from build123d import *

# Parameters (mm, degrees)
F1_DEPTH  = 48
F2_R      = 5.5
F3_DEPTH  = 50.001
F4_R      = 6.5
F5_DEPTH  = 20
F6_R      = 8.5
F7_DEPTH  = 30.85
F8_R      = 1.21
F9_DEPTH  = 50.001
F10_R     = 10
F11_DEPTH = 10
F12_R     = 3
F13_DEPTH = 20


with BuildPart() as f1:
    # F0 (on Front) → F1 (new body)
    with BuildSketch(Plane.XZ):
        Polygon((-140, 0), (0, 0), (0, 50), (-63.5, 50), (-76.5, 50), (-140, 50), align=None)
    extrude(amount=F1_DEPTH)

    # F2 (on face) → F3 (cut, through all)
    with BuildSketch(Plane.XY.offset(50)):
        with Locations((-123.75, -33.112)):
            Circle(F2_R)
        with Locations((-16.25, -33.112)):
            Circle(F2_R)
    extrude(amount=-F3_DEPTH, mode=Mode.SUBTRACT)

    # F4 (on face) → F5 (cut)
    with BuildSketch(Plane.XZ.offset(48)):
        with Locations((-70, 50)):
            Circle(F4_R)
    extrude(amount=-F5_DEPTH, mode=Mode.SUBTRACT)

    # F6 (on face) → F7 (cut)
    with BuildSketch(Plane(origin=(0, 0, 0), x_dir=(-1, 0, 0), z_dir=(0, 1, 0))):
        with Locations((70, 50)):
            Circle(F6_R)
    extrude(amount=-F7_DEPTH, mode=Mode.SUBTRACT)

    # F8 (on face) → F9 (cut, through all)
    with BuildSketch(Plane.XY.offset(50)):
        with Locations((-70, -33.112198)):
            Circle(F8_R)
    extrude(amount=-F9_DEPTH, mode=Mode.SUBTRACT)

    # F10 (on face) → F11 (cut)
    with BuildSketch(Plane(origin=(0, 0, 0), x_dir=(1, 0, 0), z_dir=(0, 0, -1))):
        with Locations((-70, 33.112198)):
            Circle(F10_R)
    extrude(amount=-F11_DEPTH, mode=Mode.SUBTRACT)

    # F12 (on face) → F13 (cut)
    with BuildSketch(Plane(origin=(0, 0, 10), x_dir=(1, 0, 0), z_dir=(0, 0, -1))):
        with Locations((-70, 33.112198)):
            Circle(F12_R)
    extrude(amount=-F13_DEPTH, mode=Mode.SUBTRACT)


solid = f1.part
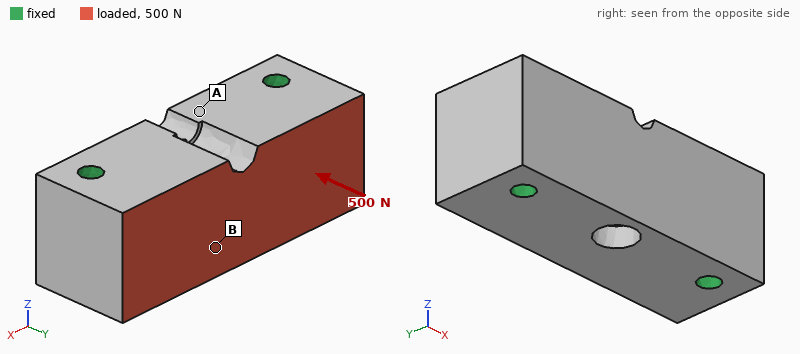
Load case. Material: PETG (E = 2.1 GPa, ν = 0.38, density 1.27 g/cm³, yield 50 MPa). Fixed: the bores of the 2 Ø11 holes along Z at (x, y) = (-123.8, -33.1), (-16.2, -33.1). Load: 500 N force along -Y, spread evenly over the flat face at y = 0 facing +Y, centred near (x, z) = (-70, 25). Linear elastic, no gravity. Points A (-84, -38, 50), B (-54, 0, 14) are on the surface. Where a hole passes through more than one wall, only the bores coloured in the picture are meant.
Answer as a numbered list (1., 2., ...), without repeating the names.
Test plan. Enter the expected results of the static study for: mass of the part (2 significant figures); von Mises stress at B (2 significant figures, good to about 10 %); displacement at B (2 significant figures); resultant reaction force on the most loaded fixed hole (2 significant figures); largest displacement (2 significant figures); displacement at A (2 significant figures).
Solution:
1. 400 g
2. 0.15 MPa
3. 5.7 µm
4. 260 N
5. 6.9 µm
6. 5.4 µm
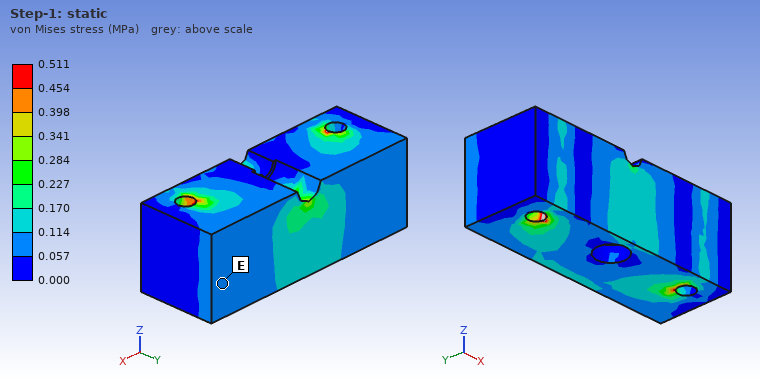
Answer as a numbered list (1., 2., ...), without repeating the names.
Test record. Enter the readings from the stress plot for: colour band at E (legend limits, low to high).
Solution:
1. 0.057 to 0.114 MPa
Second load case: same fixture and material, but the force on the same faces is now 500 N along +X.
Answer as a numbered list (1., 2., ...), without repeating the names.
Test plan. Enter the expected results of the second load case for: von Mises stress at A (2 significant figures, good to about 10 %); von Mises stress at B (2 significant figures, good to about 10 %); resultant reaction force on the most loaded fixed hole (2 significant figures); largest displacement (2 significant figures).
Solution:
1. 0.045 MPa
2. 0.13 MPa
3. 280 N
4. 7.4 µm
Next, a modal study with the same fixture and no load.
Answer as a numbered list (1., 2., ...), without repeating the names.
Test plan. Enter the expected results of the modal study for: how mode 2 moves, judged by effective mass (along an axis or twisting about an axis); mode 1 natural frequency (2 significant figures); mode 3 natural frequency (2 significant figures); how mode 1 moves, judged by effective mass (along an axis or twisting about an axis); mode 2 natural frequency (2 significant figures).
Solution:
1. along Z
2. 2400 Hz
3. 3300 Hz
4. along Y
5. 2500 Hz
